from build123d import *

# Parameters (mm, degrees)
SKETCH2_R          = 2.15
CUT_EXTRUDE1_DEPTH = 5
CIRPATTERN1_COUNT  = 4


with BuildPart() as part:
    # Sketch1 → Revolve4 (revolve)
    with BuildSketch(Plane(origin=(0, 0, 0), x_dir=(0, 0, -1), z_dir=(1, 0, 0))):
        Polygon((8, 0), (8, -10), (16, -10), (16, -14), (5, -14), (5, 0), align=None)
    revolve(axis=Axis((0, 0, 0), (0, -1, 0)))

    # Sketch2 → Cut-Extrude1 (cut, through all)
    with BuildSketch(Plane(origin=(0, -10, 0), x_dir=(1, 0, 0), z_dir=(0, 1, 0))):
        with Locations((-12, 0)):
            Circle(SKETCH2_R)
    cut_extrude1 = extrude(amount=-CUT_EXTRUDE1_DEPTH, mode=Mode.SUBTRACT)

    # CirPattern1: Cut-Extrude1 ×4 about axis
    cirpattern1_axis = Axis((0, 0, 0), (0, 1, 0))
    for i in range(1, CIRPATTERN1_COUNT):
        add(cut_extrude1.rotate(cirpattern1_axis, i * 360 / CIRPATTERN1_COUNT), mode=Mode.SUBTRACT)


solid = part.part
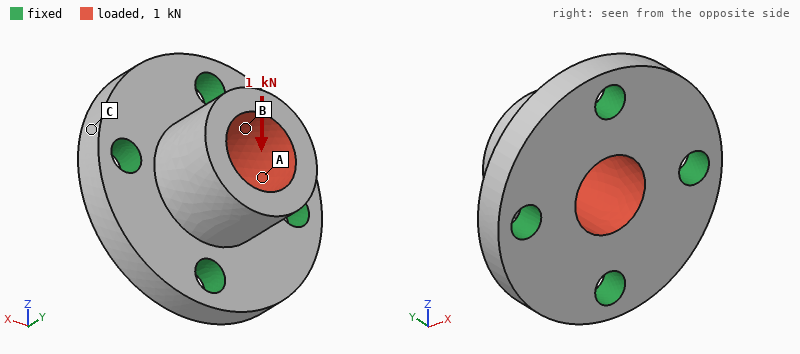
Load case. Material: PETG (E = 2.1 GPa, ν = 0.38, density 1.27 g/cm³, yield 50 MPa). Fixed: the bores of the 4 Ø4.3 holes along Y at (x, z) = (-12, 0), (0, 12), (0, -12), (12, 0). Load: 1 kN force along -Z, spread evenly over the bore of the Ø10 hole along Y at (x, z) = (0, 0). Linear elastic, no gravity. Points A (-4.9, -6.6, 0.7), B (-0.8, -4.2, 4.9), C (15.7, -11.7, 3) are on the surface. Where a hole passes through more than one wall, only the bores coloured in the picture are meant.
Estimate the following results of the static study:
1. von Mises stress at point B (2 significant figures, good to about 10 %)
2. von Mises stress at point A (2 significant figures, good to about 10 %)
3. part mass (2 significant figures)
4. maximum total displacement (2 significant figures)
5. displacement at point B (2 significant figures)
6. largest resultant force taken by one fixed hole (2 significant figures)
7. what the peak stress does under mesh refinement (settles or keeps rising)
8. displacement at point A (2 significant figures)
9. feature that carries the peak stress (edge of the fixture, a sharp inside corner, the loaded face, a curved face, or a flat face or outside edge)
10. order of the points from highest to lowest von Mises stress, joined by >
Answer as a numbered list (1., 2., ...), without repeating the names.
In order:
1. 5.8 MPa
2. 14 MPa
3. 4.9 g
4. 0.18 mm
5. 0.12 mm
6. 390 N
7. keeps rising
8. 0.082 mm
9. edge of the fixture
10. A > B > C
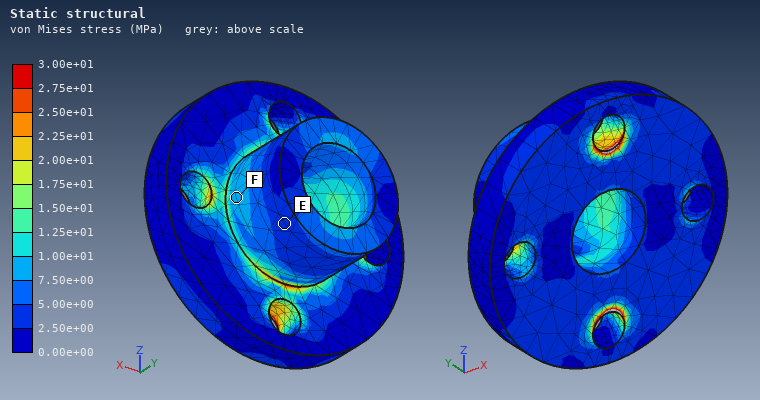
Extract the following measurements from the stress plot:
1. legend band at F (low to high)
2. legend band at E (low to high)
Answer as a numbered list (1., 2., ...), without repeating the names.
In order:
1. 7.50e+00 to 1.00e+01 MPa
2. 2.50e+00 to 5.00e+00 MPa
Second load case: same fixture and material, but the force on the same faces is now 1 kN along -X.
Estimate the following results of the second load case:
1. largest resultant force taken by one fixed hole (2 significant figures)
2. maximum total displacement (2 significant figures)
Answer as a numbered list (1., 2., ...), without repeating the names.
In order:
1. 390 N
2. 0.18 mm
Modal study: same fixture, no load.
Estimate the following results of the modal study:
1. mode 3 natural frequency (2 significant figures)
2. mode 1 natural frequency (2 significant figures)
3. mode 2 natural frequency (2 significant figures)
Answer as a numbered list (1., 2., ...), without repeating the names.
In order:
1. 12 kHz
2. 9300 Hz
3. 9400 Hz
